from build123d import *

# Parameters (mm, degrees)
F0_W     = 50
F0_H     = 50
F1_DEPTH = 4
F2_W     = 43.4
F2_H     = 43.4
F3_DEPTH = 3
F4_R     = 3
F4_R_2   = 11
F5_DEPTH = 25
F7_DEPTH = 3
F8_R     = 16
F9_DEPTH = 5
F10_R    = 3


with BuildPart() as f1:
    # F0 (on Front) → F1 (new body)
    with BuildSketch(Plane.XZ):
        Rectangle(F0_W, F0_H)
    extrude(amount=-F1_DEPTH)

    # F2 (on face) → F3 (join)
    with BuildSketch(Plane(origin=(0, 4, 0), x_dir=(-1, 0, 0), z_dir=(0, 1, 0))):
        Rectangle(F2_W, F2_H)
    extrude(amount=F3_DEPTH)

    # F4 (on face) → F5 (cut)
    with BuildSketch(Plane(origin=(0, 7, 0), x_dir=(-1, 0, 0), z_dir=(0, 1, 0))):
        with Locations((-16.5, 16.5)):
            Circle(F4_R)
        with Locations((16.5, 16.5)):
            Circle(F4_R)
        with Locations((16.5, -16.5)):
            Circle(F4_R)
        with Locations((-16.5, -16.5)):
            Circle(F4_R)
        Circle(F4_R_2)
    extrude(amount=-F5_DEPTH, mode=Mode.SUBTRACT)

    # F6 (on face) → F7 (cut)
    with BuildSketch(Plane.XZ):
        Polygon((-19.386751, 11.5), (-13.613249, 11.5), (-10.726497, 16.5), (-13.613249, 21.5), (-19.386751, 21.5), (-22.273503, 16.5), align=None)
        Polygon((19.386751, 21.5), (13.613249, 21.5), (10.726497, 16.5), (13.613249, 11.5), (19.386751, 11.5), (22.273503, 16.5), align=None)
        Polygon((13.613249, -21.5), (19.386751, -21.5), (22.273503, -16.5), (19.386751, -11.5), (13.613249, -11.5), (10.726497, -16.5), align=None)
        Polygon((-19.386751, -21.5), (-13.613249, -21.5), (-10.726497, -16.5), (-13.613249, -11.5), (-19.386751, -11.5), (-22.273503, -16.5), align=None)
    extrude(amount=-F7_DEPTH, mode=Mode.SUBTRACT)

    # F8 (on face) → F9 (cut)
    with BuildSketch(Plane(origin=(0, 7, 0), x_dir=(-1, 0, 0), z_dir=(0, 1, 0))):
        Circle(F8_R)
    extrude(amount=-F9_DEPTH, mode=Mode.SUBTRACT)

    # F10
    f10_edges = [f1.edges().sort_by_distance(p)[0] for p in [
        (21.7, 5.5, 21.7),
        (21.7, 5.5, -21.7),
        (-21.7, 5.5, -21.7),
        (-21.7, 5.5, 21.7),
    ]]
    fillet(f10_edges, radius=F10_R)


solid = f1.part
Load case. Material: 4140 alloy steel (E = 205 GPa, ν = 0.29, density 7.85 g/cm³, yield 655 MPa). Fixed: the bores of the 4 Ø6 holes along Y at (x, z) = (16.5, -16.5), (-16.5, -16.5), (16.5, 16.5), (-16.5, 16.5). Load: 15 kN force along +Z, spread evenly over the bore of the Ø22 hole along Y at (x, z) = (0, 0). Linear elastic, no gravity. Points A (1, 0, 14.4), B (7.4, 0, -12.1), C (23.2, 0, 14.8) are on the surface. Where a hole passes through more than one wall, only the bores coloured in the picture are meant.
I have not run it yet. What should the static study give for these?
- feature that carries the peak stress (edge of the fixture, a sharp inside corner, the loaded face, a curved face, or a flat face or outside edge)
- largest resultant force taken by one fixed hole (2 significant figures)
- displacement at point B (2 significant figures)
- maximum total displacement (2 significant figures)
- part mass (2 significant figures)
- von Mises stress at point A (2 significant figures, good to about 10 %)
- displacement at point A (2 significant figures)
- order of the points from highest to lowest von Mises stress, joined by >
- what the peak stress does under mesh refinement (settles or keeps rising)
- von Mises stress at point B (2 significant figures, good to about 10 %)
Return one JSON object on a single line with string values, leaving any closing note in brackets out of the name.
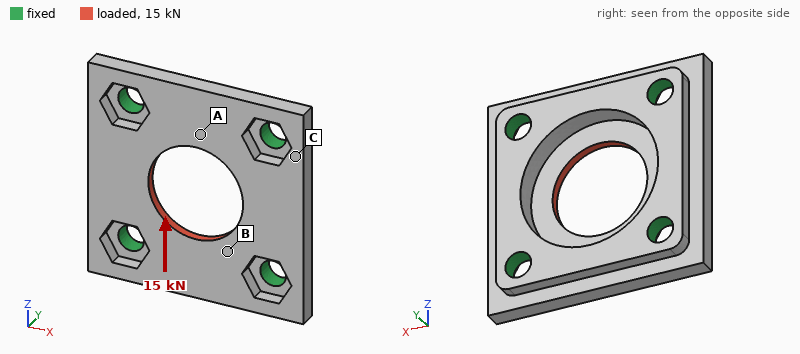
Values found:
{"feature that carries the peak stress": "edge of the fixture", "largest resultant force taken by one fixed hole": "3.8 kN", "displacement at point B": "13 µm", "maximum total displacement": "19 µm", "part mass": "73 g", "von Mises stress at point A": "92 MPa", "displacement at point A": "15 µm", "order of the points from highest to lowest von Mises stress, joined by >": "B > A > C", "what the peak stress does under mesh refinement": "keeps rising", "von Mises stress at point B": "130 MPa"}
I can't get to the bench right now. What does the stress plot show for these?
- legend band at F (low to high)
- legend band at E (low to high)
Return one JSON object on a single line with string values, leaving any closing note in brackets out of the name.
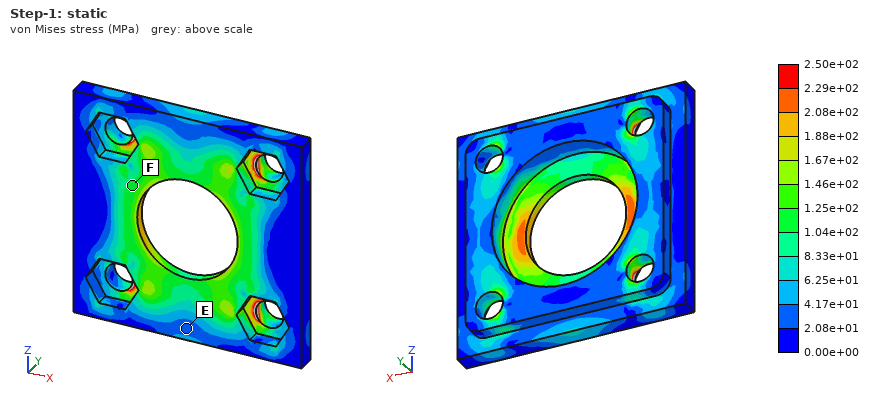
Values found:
{"legend band at F": "1.04e+02 to 1.25e+02 MPa", "legend band at E": "2.08e+01 to 4.17e+01 MPa"}
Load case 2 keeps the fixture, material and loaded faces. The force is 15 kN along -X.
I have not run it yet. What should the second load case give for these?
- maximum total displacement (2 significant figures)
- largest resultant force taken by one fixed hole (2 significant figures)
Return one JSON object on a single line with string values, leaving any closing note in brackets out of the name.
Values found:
{"maximum total displacement": "19 µm", "largest resultant force taken by one fixed hole": "3.8 kN"}
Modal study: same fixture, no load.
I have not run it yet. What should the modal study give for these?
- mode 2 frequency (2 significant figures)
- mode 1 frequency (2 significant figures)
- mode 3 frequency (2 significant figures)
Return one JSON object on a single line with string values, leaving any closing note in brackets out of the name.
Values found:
{"mode 2 frequency": "25 kHz", "mode 1 frequency": "23 kHz", "mode 3 frequency": "25 kHz"}
